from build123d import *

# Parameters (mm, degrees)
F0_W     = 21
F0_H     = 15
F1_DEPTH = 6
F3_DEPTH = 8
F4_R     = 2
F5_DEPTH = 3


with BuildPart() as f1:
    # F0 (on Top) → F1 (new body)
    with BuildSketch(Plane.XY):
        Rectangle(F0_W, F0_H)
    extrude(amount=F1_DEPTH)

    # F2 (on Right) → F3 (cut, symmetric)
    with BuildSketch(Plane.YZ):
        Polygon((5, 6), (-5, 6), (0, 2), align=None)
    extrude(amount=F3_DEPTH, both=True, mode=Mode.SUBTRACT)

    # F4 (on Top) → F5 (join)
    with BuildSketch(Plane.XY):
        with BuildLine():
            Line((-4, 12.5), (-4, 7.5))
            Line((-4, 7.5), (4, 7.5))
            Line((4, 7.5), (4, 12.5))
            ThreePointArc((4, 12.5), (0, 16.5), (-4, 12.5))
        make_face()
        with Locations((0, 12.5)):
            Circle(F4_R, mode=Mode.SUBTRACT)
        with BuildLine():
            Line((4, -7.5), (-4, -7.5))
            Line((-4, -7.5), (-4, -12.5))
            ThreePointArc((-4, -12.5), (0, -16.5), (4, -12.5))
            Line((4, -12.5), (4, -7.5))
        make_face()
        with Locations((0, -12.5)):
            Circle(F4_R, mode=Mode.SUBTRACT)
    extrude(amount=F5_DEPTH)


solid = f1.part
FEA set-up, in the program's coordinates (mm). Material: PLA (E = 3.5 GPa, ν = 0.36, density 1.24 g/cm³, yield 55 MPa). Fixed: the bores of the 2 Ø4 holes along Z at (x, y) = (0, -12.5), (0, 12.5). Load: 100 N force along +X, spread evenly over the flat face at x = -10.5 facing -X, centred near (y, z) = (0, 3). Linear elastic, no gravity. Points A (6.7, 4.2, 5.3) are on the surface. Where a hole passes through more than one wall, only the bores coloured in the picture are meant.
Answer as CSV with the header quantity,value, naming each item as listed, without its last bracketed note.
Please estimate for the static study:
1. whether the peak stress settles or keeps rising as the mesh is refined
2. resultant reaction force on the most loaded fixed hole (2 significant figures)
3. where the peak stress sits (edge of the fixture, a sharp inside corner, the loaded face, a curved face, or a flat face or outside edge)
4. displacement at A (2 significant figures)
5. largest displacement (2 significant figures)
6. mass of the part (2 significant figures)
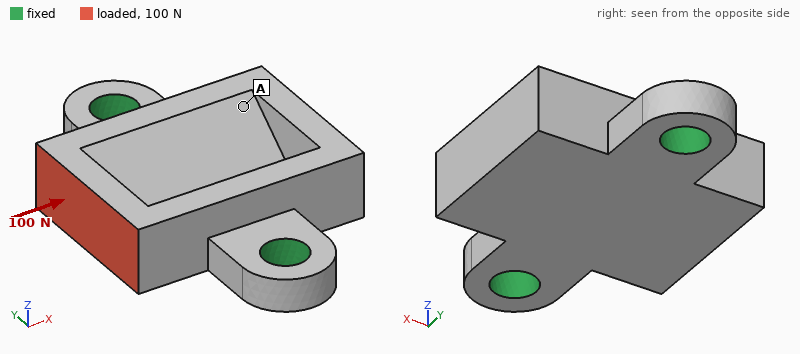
quantity,value
whether the peak stress settles or keeps rising as the mesh is refined,keeps rising
resultant reaction force on the most loaded fixed hole,50 N
where the peak stress sits,edge of the fixture
displacement at A,34 µm
largest displacement,60 µm
mass of the part,2.3 g
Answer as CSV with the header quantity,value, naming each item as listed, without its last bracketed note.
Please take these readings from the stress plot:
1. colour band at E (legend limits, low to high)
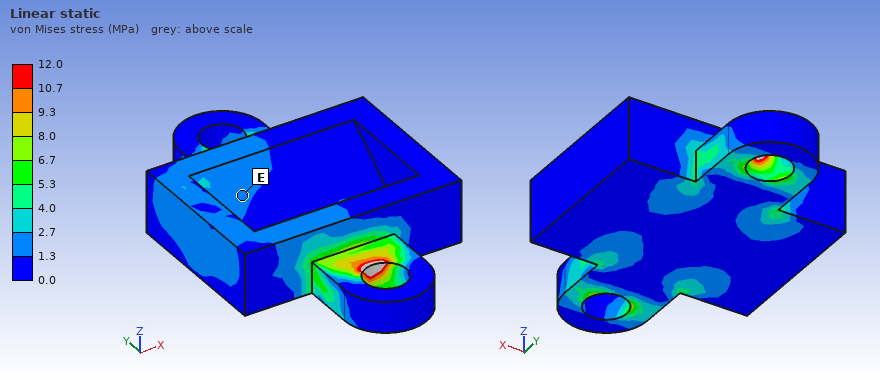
quantity,value
colour band at E,1.3 to 2.7 MPa
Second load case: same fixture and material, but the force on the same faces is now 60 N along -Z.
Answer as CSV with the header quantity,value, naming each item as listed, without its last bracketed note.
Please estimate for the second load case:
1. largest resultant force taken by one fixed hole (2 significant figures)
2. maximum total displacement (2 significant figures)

quantity,value
largest resultant force taken by one fixed hole,32 N
maximum total displacement,0.23 mm
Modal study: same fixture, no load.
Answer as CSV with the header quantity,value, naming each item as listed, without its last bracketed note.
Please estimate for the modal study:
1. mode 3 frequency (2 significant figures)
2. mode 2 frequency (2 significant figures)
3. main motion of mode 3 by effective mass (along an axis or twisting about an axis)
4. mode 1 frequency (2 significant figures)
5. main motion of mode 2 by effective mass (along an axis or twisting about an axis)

quantity,value
mode 3 frequency,11 kHz
mode 2 frequency,6000 Hz
main motion of mode 3 by effective mass,along X
mode 1 frequency,3500 Hz
main motion of mode 2 by effective mass,along Z
